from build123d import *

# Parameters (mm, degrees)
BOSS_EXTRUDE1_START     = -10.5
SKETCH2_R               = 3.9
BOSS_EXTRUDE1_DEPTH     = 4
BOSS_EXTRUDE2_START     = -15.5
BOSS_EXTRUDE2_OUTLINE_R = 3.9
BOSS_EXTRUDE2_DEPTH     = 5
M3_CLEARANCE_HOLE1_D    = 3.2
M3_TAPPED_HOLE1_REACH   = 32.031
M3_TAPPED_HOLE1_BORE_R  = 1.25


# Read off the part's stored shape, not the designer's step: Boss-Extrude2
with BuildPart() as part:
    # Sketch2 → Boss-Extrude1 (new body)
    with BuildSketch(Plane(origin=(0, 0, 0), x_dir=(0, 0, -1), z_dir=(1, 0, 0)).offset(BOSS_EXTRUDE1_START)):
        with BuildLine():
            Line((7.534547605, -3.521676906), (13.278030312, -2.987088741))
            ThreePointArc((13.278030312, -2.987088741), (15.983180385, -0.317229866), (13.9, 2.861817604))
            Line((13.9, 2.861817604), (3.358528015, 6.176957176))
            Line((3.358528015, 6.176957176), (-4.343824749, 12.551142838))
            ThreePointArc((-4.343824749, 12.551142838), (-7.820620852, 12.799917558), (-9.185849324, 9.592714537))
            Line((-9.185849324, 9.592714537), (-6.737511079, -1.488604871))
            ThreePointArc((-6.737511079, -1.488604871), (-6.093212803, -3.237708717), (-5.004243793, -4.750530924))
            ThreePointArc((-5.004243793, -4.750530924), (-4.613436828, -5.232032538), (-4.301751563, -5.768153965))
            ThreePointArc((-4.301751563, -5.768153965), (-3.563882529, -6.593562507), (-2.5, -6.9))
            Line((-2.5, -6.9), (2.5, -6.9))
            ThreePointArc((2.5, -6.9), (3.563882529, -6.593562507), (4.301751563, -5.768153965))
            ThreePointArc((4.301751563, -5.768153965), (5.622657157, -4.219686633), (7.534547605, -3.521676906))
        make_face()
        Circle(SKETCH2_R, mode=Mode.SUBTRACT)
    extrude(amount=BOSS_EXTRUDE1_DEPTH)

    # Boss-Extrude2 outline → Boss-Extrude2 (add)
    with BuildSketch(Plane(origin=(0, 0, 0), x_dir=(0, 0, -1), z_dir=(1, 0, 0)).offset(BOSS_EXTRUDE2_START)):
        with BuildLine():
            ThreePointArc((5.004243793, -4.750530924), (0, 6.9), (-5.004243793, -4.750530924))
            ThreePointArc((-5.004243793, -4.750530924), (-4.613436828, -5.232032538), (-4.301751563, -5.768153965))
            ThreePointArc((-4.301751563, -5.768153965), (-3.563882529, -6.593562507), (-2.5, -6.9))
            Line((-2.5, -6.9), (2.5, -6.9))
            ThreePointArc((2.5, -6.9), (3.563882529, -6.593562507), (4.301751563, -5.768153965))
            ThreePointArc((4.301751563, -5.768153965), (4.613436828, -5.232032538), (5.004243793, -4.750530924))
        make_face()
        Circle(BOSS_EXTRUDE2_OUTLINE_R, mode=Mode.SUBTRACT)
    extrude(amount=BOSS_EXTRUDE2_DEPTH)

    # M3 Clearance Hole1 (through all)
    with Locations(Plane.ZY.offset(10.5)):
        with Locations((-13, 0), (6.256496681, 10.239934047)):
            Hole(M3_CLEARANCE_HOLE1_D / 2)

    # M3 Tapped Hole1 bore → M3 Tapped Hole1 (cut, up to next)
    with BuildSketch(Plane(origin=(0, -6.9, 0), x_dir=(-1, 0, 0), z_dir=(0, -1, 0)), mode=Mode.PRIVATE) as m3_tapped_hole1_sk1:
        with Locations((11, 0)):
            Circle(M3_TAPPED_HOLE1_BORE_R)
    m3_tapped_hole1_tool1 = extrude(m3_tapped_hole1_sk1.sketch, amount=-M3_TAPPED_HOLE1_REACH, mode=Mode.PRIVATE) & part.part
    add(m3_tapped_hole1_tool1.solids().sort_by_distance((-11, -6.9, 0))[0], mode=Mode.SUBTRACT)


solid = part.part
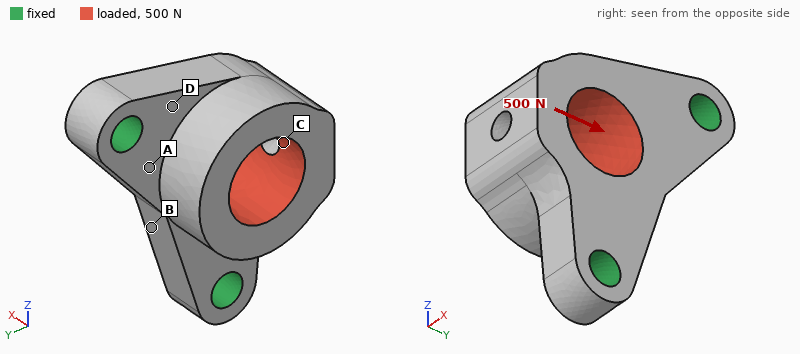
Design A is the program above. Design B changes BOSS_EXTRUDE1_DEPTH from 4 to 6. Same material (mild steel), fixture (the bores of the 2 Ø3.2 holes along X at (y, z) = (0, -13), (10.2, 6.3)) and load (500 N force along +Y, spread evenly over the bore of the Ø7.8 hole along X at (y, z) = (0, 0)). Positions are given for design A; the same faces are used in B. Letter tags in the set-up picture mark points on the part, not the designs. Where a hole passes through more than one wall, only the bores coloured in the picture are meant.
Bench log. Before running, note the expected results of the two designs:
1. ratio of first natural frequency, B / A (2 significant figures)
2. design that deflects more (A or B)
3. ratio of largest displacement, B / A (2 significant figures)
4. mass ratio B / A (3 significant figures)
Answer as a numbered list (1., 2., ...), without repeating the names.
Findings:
1. 1.4
2. A
3. 0.45
4. 1.32
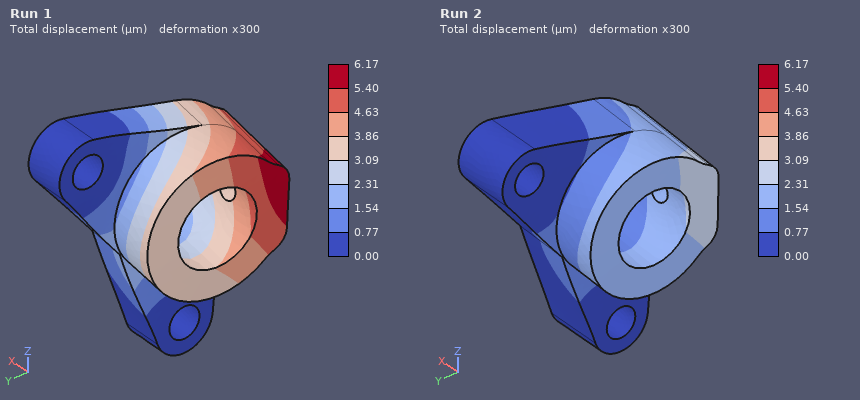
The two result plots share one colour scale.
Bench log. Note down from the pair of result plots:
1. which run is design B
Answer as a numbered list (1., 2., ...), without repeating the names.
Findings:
1. Run 2
